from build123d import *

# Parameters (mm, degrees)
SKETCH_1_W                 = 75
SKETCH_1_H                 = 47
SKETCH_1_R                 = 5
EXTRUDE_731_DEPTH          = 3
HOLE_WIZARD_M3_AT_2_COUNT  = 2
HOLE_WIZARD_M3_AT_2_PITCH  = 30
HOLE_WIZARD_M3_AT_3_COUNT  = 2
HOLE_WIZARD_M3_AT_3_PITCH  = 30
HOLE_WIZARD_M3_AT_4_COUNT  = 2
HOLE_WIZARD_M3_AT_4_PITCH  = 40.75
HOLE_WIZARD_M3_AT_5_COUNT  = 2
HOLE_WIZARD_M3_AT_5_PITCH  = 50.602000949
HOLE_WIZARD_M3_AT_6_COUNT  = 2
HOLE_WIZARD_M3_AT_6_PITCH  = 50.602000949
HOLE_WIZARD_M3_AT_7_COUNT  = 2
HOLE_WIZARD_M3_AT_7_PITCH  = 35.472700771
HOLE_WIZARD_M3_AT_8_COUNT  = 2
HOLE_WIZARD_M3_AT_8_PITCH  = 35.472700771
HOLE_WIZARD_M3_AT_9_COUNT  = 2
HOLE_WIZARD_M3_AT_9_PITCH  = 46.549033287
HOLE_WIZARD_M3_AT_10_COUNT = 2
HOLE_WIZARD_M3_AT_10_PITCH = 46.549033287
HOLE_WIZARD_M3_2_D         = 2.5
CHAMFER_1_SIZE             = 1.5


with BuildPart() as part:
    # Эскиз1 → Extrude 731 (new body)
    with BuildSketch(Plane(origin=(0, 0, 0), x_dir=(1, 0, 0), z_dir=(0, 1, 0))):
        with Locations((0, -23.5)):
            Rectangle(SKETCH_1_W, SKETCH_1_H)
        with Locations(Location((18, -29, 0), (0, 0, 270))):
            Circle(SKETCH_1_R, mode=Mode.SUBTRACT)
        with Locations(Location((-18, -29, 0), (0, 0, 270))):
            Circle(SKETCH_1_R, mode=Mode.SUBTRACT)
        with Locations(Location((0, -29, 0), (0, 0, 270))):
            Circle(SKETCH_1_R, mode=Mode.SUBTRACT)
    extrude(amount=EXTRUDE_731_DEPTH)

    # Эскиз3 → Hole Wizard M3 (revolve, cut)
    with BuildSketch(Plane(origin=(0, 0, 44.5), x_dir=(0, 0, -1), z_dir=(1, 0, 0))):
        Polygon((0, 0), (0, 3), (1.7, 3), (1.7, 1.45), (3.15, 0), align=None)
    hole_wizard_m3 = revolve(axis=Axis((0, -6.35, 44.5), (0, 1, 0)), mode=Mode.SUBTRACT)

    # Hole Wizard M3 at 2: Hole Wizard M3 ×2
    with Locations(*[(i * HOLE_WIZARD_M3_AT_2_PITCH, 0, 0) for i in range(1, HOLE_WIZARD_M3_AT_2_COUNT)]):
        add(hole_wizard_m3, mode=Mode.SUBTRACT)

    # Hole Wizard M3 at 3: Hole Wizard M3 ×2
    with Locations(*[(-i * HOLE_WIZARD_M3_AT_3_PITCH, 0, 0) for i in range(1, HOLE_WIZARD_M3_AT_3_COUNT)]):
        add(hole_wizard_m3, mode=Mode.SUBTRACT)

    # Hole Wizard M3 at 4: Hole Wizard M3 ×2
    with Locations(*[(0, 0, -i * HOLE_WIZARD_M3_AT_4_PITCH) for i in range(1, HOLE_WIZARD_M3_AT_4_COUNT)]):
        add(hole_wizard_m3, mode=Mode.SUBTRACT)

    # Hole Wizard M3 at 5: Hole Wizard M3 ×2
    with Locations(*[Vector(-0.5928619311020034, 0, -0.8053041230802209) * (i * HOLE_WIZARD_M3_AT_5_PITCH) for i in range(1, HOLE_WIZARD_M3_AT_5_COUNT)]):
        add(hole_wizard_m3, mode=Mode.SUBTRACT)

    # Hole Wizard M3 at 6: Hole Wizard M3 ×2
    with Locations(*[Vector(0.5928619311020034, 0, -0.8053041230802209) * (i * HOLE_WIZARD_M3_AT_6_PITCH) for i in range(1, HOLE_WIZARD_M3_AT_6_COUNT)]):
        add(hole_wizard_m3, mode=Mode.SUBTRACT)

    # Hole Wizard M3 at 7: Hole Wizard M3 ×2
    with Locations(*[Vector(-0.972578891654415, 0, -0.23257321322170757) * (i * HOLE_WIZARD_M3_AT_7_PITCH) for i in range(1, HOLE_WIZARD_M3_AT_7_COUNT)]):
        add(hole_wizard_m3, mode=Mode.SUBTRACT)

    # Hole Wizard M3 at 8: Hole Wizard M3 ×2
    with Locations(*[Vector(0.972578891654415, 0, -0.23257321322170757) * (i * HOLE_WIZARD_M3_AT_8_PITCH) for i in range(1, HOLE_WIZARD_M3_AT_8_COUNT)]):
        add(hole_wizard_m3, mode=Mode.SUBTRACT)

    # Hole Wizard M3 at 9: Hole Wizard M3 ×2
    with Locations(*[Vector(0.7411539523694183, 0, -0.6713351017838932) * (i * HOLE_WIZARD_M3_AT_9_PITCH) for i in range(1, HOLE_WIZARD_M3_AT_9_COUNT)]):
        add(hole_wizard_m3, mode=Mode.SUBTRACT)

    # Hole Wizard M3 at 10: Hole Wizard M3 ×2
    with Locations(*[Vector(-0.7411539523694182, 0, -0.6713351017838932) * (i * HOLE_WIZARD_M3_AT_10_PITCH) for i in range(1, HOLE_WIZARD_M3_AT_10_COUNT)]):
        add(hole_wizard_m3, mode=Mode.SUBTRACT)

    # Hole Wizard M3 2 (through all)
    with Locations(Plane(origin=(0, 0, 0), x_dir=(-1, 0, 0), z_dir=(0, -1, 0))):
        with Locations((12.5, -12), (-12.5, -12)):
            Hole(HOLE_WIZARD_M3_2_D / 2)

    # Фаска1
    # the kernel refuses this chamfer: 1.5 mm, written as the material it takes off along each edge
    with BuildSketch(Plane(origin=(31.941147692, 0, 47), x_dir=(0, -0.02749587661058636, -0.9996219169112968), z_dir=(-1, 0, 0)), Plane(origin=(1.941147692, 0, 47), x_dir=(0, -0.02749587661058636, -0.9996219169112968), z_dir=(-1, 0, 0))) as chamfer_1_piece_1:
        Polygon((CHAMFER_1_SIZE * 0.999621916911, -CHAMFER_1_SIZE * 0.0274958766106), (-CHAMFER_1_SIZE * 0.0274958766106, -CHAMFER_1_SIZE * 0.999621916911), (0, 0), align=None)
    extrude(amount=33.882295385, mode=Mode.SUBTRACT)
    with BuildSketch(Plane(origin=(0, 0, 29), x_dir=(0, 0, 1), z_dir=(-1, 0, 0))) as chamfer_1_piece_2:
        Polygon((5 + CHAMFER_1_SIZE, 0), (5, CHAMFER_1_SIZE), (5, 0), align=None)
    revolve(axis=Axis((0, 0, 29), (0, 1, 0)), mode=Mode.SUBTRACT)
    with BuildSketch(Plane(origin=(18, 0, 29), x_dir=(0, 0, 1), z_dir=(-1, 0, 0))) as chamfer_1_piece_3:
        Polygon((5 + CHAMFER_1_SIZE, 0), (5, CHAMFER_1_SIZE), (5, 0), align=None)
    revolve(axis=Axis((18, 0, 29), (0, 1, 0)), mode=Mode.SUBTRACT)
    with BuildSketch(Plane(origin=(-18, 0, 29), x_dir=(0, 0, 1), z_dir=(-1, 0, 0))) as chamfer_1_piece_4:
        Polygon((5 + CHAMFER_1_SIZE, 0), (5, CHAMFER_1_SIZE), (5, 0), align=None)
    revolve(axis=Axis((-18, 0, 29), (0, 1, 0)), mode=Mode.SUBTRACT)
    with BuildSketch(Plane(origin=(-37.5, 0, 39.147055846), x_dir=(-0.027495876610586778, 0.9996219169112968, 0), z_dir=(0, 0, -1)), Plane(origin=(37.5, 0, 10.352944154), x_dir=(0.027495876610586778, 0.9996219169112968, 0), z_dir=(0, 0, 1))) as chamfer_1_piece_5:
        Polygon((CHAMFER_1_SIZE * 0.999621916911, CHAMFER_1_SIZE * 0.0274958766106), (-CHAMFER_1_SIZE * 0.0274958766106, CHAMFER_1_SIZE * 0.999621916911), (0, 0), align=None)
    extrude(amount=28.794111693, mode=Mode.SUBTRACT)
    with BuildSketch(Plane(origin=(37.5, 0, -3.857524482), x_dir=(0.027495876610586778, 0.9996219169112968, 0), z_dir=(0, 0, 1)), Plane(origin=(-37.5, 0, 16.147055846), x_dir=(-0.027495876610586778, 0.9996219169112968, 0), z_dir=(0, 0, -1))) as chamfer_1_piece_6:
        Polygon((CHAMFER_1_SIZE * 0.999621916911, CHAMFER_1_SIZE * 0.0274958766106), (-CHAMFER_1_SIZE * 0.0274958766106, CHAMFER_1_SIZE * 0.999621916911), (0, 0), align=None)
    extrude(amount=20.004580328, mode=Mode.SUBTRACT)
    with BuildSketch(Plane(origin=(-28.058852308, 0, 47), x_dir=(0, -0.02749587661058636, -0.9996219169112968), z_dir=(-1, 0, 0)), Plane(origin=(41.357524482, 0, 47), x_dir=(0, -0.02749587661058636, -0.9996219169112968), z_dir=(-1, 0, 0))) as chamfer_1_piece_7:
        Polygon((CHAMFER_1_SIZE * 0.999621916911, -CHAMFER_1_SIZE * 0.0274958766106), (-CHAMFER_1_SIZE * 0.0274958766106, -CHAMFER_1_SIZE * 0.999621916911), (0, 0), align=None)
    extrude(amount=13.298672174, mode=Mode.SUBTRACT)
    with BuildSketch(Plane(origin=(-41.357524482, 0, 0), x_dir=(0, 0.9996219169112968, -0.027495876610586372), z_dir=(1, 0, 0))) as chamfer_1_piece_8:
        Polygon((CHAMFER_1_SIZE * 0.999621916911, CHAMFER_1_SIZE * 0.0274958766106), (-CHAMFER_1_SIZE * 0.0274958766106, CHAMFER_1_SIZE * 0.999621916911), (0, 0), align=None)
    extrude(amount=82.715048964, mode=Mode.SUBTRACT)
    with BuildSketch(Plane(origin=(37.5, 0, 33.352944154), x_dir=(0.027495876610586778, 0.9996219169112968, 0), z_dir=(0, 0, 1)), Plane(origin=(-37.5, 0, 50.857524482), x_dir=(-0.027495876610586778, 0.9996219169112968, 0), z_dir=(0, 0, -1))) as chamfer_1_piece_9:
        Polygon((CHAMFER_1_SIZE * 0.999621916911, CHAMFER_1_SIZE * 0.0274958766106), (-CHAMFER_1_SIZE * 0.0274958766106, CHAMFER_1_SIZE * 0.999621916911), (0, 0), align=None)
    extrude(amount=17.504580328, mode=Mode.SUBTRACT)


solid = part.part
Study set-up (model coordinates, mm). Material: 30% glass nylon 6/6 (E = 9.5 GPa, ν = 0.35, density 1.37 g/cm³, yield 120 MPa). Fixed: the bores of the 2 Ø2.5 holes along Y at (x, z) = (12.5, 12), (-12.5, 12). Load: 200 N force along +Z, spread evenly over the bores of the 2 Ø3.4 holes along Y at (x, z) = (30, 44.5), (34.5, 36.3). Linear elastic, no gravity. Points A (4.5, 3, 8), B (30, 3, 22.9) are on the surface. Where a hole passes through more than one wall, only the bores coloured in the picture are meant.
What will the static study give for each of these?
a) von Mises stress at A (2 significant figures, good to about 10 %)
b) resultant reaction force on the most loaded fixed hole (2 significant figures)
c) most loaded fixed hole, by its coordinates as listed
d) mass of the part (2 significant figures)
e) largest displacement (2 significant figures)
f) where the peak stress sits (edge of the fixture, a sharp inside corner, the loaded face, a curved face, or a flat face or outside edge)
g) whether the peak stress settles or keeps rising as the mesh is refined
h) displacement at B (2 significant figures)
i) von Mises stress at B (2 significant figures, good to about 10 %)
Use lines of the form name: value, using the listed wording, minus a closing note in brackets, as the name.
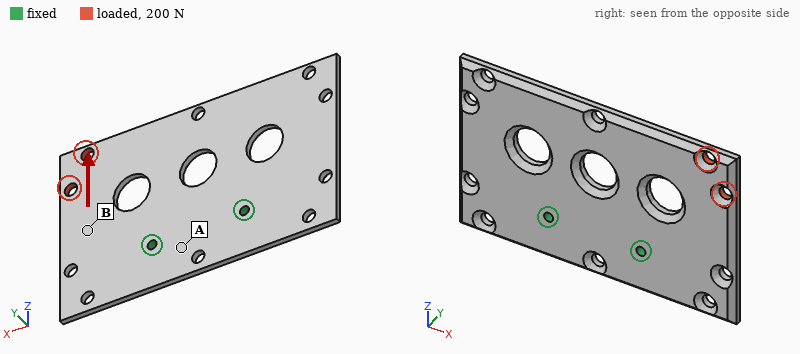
von Mises stress at A: 2.8 MPa
resultant reaction force on the most loaded fixed hole: 350 N
most loaded fixed hole, by its coordinates as listed: (12.5, 12)
mass of the part: 12 g
largest displacement: 0.19 mm
where the peak stress sits: edge of the fixture
whether the peak stress settles or keeps rising as the mesh is refined: keeps rising
displacement at B: 0.049 mm
von Mises stress at B: 6.2 MPa
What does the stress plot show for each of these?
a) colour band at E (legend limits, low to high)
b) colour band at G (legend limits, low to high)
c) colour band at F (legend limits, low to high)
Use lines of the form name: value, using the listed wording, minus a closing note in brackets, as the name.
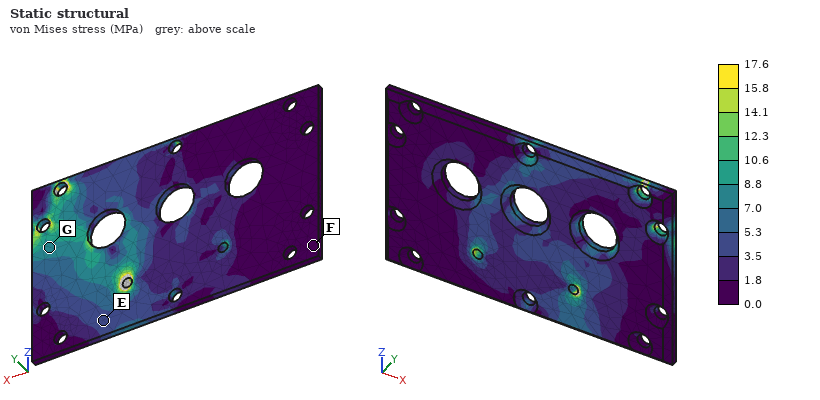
colour band at E: 3.5 to 5.3 MPa
colour band at G: 7.0 to 8.8 MPa
colour band at F: 0.0 to 1.8 MPa
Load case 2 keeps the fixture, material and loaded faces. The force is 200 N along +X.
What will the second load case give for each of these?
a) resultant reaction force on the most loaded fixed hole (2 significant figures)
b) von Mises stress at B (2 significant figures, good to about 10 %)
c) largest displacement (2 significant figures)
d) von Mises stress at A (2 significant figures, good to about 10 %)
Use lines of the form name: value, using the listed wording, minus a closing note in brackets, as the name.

resultant reaction force on the most loaded fixed hole: 240 N
von Mises stress at B: 3.5 MPa
largest displacement: 0.15 mm
von Mises stress at A: 2.8 MPa
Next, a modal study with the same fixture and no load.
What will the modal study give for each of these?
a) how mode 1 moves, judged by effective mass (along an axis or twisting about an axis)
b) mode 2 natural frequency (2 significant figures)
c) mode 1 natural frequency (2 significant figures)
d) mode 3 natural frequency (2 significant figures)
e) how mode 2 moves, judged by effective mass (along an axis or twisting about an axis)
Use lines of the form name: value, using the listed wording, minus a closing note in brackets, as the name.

how mode 1 moves, judged by effective mass: along Y
mode 2 natural frequency: 1000 Hz
mode 1 natural frequency: 830 Hz
mode 3 natural frequency: 1700 Hz
how mode 2 moves, judged by effective mass: twisting about Z
